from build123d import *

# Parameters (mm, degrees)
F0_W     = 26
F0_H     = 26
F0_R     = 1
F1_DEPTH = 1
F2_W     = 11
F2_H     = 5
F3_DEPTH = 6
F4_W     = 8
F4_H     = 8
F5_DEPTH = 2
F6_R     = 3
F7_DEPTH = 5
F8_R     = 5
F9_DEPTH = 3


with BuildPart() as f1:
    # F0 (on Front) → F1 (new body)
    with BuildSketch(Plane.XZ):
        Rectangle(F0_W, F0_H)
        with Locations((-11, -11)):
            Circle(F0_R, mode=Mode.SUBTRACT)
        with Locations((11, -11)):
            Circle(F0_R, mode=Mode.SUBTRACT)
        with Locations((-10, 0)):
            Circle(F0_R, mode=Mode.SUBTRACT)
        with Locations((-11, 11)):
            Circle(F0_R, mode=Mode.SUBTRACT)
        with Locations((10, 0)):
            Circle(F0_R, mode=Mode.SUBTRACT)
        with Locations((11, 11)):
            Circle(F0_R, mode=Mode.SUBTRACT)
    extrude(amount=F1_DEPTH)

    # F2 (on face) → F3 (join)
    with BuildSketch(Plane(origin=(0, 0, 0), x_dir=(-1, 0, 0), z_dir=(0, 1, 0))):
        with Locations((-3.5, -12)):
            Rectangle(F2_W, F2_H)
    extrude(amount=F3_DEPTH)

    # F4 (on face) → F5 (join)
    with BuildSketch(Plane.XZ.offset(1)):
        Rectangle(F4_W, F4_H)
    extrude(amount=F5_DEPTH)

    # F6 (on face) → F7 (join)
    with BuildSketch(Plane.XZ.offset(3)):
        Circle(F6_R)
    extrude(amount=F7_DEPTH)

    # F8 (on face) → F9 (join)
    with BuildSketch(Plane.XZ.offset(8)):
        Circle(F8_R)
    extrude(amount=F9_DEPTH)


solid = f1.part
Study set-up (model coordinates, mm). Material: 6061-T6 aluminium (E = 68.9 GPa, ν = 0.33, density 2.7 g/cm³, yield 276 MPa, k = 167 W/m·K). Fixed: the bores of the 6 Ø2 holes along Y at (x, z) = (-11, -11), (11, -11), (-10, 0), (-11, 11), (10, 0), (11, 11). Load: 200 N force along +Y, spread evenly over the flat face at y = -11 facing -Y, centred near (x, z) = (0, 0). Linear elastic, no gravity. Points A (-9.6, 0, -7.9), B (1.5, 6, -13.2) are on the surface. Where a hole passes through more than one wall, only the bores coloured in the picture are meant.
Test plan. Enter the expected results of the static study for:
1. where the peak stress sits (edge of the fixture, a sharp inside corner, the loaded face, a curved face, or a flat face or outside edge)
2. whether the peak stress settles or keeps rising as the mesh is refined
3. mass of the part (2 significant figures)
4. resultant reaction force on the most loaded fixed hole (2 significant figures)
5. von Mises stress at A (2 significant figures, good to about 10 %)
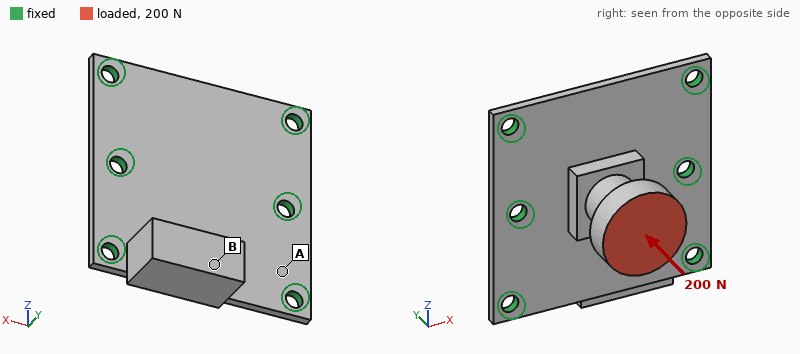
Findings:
edge of the fixture
keeps rising
4.0 g
84 N
27 MPa
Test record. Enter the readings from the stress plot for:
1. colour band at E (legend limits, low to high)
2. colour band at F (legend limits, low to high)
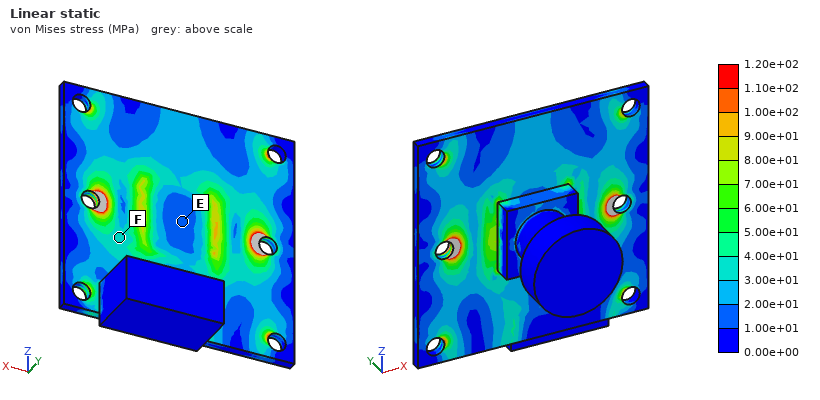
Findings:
1.00e+01 to 2.00e+01 MPa
3.00e+01 to 4.00e+01 MPa
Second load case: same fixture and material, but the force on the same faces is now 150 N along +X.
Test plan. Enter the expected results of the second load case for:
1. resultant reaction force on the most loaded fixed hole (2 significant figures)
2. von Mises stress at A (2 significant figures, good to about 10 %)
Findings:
99 N
21 MPa
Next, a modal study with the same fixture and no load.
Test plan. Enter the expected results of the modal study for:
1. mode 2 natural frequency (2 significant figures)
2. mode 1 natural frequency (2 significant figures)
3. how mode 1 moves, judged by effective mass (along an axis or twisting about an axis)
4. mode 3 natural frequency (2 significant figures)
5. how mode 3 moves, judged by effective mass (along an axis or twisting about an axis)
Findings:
7900 Hz
6400 Hz
along Z
9000 Hz
along Y
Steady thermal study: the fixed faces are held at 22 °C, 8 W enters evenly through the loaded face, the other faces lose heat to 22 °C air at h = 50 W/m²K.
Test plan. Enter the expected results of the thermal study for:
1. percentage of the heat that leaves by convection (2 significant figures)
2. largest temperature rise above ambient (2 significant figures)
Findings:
7.1 %
24 K
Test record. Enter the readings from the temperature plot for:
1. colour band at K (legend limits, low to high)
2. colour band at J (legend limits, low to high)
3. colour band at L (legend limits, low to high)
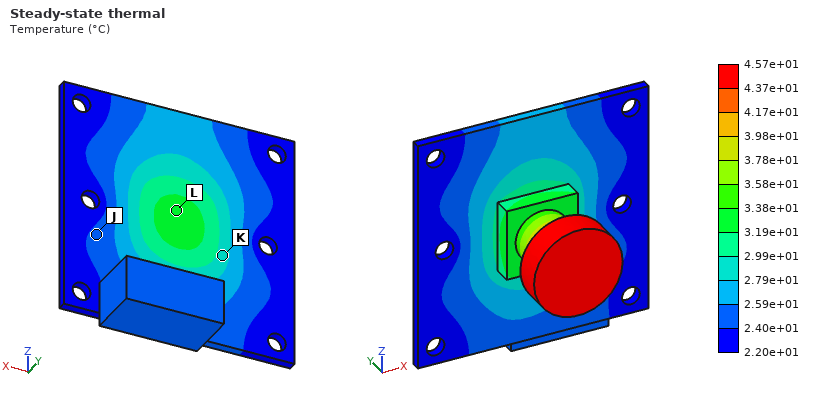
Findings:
2.79e+01 to 2.99e+01 °C
2.40e+01 to 2.59e+01 °C
3.19e+01 to 3.38e+01 °C
